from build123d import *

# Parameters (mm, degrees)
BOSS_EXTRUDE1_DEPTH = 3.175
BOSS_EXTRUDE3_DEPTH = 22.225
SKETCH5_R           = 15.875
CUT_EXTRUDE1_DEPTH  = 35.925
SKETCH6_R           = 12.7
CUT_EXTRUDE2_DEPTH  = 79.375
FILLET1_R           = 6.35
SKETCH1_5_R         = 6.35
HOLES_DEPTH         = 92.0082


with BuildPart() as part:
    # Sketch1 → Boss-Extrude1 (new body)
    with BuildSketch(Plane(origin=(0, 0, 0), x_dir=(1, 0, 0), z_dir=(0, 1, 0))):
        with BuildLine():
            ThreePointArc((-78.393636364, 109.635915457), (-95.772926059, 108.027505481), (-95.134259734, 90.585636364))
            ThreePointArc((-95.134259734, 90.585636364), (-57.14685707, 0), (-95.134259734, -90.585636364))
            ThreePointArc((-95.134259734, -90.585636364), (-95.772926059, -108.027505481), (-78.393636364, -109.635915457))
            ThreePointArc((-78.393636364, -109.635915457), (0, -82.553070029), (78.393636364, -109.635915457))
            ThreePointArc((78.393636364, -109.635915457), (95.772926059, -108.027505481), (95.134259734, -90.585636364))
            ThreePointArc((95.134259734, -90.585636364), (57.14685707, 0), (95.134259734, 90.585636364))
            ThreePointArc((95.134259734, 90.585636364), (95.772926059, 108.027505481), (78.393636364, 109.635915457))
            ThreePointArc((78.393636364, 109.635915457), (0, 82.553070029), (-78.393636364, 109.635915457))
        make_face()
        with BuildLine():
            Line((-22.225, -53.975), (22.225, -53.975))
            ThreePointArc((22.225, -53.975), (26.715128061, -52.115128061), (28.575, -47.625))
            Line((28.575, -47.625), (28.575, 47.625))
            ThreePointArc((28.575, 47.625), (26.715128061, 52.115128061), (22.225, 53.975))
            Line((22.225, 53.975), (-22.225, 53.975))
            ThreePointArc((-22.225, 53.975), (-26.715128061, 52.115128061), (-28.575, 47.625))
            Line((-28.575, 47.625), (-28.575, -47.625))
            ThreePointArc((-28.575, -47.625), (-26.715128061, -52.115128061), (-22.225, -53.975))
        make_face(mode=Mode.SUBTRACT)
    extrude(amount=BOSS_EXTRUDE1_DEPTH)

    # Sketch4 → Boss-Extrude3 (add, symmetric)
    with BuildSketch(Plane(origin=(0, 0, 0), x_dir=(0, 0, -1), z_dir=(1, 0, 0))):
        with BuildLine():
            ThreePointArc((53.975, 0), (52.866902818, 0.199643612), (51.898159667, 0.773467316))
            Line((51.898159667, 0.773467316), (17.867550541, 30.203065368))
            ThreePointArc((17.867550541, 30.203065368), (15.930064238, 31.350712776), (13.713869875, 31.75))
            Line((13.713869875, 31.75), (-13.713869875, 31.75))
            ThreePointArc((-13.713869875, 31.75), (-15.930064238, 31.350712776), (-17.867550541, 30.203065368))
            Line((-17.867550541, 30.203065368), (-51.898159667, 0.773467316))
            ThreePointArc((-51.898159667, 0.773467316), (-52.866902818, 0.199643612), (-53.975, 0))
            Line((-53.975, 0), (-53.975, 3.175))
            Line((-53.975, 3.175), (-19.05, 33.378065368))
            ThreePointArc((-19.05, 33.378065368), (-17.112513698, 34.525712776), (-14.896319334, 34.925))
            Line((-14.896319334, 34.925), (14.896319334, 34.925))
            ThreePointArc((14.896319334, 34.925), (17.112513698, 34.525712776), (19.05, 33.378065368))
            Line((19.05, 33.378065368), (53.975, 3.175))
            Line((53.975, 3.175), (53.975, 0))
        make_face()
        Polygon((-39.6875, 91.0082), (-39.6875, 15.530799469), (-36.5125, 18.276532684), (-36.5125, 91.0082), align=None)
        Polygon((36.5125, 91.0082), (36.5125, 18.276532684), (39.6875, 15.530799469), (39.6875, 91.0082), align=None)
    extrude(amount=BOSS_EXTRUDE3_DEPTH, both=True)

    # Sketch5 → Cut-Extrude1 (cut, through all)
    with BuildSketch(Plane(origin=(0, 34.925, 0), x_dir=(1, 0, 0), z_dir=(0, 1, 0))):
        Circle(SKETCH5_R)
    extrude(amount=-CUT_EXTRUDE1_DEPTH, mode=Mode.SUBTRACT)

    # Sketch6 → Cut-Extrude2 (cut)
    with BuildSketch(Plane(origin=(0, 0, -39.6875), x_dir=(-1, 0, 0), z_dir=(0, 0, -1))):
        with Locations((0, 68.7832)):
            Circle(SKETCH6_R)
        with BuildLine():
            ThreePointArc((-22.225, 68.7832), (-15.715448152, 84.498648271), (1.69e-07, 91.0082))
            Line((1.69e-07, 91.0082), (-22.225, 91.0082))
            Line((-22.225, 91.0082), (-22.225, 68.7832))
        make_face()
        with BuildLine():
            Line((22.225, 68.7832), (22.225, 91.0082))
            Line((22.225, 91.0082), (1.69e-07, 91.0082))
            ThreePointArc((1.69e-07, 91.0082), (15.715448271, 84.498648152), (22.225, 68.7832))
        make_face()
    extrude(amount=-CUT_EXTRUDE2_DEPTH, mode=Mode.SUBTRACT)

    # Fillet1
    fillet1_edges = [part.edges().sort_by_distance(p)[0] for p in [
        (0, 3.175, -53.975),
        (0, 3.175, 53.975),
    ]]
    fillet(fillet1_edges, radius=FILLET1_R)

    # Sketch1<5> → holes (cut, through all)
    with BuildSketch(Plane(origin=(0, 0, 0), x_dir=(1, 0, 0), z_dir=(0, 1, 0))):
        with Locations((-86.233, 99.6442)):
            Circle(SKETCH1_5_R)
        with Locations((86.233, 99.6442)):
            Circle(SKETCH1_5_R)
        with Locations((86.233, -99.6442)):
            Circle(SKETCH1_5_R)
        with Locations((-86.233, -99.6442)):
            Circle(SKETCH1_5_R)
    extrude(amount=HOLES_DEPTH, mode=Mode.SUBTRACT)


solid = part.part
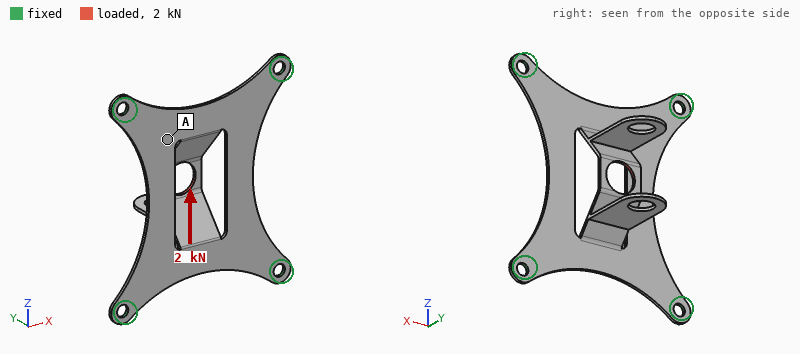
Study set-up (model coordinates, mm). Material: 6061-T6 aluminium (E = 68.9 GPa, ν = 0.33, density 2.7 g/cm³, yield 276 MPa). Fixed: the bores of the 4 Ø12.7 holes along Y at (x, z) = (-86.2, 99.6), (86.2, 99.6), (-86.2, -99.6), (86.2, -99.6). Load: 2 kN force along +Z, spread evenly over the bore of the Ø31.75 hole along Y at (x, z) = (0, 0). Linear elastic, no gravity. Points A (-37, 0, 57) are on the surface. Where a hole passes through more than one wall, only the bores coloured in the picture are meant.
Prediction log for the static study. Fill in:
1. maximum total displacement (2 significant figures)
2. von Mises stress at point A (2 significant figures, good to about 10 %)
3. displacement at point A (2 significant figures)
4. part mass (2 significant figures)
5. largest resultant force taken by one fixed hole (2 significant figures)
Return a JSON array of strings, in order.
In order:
["2.2 mm", "40 MPa", "0.63 mm", "260 g", "720 N"]
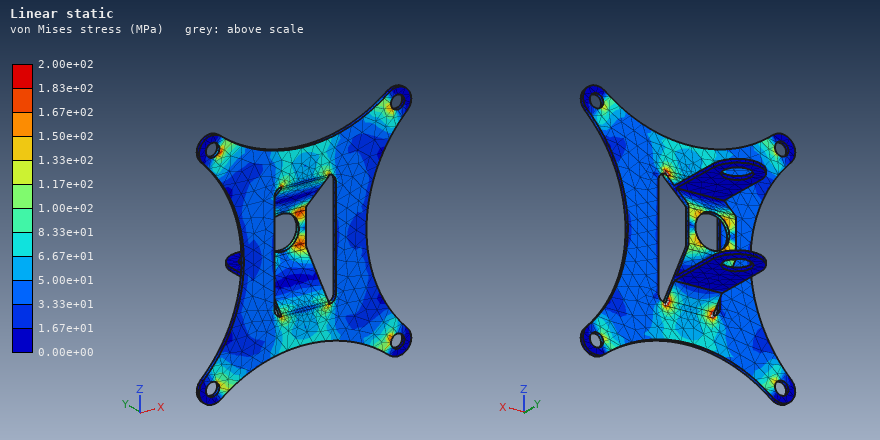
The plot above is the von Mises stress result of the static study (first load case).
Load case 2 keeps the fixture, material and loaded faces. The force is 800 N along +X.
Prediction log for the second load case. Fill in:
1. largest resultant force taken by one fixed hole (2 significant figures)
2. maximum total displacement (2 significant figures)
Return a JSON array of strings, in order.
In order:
["260 N", "1.6 mm"]
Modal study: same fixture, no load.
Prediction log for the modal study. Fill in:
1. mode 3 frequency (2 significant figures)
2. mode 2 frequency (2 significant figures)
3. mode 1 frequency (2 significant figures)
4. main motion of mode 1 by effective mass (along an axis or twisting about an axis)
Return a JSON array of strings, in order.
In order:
["410 Hz", "390 Hz", "260 Hz", "along Y"]
